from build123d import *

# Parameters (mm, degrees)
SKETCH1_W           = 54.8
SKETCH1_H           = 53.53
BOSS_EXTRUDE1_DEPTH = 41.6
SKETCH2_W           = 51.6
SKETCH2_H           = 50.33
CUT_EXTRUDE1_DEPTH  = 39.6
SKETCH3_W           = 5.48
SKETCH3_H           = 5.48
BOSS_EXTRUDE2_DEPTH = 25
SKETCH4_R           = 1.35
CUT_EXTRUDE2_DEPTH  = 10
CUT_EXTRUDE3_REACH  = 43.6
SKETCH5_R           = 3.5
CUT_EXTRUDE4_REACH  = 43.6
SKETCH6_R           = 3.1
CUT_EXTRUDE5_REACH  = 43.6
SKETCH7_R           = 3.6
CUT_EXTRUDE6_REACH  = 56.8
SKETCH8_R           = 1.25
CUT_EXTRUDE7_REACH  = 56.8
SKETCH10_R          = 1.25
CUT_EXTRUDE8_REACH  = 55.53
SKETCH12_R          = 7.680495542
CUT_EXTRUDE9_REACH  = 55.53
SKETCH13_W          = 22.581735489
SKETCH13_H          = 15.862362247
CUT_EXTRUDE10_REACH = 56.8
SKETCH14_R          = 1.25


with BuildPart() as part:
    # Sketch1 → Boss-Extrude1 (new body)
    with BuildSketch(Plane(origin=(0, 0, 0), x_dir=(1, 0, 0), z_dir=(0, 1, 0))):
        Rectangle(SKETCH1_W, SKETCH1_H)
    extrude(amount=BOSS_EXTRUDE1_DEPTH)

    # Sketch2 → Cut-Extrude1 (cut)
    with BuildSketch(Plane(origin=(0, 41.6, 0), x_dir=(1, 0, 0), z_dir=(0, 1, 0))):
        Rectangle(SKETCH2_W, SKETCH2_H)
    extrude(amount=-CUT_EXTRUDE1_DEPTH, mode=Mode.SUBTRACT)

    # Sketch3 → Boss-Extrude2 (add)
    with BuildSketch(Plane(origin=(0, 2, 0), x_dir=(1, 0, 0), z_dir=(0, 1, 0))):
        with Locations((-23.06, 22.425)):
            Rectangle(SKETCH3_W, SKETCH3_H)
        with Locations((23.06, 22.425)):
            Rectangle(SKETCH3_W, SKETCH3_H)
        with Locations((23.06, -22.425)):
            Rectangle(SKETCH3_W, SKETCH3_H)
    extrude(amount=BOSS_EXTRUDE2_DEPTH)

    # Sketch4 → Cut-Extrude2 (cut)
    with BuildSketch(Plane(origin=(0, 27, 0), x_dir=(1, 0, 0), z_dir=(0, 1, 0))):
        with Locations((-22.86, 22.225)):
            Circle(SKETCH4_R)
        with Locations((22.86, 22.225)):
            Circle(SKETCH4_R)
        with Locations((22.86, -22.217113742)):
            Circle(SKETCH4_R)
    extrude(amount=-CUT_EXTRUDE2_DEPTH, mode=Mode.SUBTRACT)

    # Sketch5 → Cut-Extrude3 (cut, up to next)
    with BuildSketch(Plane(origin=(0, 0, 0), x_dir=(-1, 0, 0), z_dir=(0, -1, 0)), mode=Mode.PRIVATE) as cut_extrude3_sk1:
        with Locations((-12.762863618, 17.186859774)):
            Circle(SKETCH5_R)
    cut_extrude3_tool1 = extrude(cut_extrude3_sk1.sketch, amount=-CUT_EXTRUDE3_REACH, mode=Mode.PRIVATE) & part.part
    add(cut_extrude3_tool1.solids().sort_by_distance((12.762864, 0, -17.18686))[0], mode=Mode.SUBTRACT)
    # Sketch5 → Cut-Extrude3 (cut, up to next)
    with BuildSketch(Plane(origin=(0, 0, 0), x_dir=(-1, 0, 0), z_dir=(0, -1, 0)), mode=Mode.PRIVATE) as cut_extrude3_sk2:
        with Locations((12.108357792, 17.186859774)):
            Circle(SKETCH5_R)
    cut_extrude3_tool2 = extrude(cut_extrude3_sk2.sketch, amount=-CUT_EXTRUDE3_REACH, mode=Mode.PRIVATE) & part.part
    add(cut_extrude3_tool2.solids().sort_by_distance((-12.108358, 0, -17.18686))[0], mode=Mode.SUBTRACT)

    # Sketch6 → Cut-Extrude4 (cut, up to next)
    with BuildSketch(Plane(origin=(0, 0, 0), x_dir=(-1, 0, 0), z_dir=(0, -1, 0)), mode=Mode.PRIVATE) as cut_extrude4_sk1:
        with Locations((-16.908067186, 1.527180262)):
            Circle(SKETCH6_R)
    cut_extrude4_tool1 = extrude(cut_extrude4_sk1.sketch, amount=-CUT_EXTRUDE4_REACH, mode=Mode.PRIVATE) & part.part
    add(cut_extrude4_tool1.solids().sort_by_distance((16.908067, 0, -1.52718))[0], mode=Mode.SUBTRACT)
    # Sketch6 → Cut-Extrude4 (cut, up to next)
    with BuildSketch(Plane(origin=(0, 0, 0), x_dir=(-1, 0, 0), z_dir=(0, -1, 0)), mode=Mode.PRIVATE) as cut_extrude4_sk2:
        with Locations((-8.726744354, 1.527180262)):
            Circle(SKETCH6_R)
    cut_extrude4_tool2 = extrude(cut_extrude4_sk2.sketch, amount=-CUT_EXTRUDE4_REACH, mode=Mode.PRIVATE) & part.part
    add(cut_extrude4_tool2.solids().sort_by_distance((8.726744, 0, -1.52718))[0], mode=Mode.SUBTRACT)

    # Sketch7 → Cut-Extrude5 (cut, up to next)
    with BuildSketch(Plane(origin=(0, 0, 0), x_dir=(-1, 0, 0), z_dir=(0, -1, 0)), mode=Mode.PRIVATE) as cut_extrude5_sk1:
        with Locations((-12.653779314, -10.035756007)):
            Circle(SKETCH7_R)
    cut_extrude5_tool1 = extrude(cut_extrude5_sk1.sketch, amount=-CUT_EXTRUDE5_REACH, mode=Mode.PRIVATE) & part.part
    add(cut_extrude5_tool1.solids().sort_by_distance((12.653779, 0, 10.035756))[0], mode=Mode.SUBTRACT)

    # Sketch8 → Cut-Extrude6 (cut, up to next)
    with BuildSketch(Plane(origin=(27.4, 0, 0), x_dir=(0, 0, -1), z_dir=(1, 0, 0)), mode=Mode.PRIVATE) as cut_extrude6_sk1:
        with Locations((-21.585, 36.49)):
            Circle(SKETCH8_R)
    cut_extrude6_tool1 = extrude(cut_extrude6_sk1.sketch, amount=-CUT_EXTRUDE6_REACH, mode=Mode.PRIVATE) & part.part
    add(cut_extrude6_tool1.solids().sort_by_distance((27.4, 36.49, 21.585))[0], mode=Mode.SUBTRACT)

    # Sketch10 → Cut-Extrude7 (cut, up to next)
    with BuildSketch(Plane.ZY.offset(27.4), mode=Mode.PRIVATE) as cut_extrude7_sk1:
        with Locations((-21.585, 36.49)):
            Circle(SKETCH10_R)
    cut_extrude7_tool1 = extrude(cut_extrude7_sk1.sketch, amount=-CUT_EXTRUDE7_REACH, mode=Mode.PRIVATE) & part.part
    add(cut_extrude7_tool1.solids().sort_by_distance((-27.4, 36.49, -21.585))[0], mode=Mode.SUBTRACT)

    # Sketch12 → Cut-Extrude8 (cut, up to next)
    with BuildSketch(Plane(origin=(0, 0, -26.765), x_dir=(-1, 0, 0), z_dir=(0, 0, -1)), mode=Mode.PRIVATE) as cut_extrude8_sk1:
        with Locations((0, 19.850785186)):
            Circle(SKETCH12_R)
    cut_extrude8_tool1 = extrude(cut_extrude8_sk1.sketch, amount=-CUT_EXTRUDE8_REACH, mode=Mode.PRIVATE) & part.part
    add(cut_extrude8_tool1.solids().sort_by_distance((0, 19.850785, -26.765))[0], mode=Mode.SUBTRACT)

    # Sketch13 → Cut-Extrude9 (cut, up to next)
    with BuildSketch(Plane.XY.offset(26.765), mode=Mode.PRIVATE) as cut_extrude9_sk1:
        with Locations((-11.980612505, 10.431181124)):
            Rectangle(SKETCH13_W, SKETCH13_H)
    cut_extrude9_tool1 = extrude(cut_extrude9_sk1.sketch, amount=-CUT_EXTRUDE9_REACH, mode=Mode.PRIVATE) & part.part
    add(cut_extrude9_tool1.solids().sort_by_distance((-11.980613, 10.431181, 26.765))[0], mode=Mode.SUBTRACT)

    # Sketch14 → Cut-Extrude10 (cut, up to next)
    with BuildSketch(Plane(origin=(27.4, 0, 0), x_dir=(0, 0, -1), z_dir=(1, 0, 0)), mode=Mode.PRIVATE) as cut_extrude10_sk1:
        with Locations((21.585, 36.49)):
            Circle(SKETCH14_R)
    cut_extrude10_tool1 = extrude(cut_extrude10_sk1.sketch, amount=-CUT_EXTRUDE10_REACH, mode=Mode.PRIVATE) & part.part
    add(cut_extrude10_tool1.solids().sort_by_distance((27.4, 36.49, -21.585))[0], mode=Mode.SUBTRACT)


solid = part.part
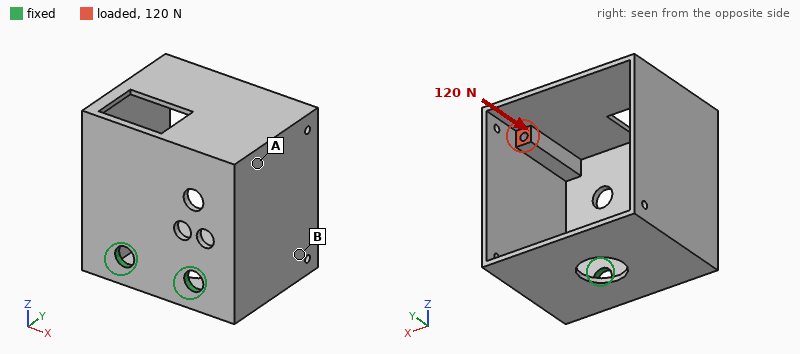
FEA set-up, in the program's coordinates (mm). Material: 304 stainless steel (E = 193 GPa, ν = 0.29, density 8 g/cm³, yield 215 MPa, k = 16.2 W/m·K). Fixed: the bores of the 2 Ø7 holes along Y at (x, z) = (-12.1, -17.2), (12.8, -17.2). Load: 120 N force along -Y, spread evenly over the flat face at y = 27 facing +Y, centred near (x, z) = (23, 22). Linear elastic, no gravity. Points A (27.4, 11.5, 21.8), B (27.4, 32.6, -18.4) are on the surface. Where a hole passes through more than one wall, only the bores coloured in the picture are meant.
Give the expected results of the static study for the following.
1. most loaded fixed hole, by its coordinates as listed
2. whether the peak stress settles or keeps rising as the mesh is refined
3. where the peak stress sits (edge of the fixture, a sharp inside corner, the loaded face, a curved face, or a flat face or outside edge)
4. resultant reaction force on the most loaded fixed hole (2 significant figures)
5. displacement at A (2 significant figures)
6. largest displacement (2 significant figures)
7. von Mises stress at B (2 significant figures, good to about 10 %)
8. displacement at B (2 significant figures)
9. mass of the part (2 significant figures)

(12.8, -17.2)
keeps rising
edge of the fixture
130 N
0.10 mm
0.15 mm
14 MPa
0.071 mm
160 g
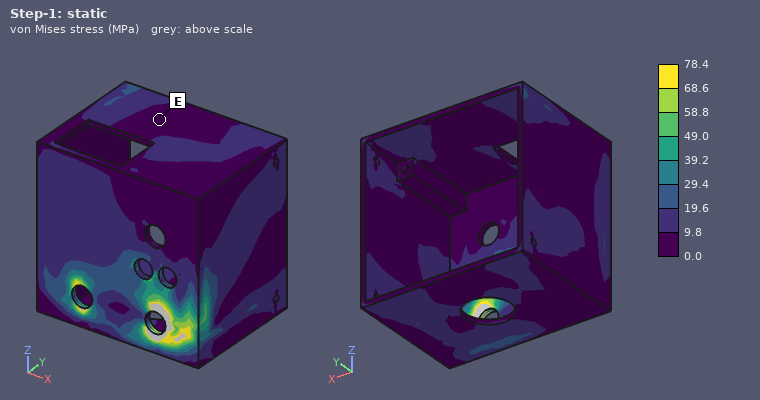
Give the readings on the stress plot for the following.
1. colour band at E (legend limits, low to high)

0.0 to 9.8 MPa
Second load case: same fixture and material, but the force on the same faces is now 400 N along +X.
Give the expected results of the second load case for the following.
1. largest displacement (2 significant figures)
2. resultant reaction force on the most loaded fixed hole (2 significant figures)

0.27 mm
600 N
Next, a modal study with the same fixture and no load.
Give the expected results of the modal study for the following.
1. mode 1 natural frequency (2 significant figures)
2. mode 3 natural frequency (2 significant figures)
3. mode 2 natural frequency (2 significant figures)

660 Hz
2400 Hz
910 Hz
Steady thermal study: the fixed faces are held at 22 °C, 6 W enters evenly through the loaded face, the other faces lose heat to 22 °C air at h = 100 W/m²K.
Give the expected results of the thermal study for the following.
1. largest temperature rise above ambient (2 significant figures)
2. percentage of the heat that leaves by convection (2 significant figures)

82 K
99 %
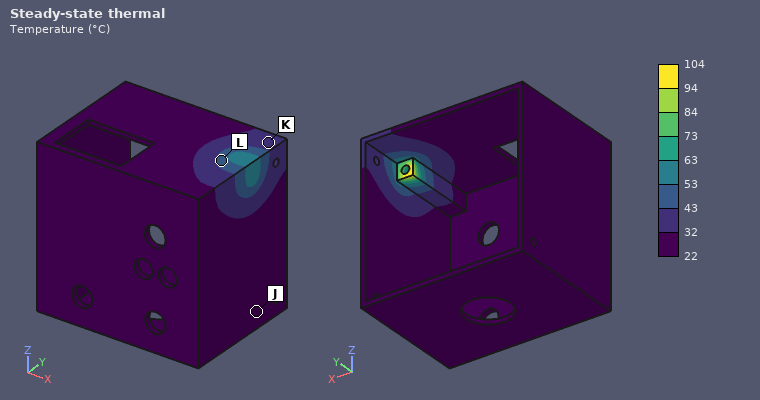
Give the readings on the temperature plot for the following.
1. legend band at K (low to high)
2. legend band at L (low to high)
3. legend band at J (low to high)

32 to 43 °C
43 to 53 °C
22 to 32 °C
